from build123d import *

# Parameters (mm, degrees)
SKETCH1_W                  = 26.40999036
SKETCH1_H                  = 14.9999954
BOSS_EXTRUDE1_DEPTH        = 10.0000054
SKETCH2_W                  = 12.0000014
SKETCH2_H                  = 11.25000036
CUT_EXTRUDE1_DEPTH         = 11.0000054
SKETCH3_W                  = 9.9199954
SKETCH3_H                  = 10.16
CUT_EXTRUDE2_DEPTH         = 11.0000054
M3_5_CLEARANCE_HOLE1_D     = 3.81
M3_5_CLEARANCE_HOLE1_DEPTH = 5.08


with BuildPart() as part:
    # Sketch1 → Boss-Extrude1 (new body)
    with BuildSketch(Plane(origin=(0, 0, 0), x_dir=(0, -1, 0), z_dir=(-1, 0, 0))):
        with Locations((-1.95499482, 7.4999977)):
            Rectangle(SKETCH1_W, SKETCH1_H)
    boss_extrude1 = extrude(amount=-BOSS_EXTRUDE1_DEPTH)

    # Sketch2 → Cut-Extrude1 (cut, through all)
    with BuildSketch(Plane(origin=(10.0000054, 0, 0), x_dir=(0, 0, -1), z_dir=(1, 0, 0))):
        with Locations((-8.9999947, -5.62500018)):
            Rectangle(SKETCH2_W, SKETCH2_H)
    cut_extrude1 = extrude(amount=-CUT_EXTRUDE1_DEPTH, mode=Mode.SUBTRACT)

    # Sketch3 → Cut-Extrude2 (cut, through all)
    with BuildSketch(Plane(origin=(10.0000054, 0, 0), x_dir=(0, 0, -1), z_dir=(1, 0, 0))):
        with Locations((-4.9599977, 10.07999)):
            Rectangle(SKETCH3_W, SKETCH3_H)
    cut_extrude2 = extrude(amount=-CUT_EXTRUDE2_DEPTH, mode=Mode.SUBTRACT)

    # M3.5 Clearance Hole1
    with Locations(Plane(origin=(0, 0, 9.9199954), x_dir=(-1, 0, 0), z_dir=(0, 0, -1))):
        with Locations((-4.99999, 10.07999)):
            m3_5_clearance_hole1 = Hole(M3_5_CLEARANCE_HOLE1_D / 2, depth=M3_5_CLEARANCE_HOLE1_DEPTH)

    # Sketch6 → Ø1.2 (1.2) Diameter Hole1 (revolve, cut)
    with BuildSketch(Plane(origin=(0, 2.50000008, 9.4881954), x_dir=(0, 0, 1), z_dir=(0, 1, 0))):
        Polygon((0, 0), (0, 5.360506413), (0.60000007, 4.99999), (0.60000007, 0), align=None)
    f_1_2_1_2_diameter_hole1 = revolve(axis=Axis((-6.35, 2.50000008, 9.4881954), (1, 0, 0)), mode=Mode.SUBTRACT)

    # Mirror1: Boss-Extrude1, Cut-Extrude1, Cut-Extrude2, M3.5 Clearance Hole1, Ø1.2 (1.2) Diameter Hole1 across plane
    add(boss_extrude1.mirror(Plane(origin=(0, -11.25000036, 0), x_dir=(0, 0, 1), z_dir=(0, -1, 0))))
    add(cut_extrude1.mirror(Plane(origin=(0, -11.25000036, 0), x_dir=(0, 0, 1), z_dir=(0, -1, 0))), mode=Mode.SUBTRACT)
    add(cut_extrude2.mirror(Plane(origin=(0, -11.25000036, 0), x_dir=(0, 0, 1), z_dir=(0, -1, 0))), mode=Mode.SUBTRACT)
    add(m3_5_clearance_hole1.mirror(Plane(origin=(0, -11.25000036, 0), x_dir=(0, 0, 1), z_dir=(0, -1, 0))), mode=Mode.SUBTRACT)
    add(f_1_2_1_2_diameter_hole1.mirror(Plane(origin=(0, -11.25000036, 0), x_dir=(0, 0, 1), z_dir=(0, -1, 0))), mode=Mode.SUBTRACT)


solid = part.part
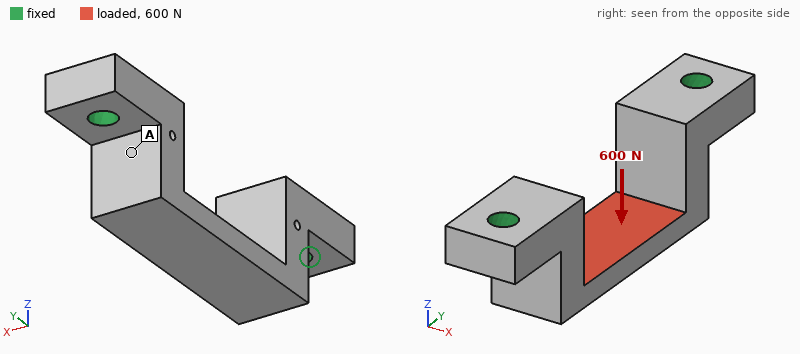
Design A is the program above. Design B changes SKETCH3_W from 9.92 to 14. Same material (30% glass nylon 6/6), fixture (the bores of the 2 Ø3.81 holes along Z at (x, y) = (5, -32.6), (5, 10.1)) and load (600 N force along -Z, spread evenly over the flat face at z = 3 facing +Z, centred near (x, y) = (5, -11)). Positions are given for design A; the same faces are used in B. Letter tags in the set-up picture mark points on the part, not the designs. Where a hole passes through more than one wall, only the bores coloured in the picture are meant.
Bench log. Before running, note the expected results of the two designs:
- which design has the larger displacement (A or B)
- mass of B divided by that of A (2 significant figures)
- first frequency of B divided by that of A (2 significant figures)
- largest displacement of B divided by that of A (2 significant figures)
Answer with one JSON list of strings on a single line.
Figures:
["B", "0.88", "0.61", "1.1"]
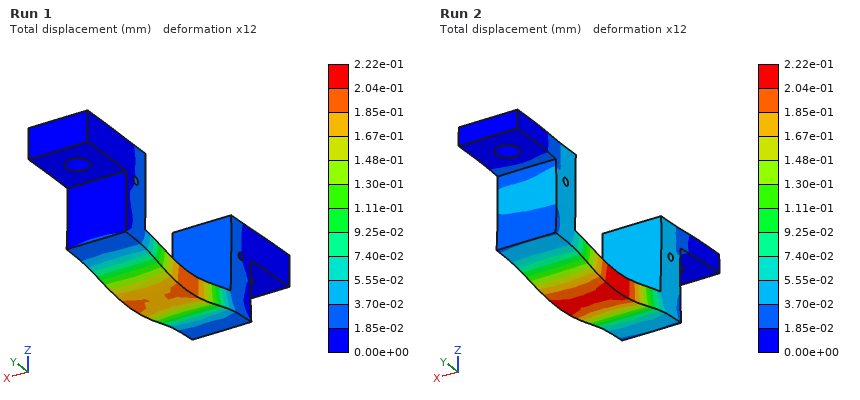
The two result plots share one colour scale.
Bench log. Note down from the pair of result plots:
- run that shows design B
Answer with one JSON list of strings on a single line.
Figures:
["Run 2"]
